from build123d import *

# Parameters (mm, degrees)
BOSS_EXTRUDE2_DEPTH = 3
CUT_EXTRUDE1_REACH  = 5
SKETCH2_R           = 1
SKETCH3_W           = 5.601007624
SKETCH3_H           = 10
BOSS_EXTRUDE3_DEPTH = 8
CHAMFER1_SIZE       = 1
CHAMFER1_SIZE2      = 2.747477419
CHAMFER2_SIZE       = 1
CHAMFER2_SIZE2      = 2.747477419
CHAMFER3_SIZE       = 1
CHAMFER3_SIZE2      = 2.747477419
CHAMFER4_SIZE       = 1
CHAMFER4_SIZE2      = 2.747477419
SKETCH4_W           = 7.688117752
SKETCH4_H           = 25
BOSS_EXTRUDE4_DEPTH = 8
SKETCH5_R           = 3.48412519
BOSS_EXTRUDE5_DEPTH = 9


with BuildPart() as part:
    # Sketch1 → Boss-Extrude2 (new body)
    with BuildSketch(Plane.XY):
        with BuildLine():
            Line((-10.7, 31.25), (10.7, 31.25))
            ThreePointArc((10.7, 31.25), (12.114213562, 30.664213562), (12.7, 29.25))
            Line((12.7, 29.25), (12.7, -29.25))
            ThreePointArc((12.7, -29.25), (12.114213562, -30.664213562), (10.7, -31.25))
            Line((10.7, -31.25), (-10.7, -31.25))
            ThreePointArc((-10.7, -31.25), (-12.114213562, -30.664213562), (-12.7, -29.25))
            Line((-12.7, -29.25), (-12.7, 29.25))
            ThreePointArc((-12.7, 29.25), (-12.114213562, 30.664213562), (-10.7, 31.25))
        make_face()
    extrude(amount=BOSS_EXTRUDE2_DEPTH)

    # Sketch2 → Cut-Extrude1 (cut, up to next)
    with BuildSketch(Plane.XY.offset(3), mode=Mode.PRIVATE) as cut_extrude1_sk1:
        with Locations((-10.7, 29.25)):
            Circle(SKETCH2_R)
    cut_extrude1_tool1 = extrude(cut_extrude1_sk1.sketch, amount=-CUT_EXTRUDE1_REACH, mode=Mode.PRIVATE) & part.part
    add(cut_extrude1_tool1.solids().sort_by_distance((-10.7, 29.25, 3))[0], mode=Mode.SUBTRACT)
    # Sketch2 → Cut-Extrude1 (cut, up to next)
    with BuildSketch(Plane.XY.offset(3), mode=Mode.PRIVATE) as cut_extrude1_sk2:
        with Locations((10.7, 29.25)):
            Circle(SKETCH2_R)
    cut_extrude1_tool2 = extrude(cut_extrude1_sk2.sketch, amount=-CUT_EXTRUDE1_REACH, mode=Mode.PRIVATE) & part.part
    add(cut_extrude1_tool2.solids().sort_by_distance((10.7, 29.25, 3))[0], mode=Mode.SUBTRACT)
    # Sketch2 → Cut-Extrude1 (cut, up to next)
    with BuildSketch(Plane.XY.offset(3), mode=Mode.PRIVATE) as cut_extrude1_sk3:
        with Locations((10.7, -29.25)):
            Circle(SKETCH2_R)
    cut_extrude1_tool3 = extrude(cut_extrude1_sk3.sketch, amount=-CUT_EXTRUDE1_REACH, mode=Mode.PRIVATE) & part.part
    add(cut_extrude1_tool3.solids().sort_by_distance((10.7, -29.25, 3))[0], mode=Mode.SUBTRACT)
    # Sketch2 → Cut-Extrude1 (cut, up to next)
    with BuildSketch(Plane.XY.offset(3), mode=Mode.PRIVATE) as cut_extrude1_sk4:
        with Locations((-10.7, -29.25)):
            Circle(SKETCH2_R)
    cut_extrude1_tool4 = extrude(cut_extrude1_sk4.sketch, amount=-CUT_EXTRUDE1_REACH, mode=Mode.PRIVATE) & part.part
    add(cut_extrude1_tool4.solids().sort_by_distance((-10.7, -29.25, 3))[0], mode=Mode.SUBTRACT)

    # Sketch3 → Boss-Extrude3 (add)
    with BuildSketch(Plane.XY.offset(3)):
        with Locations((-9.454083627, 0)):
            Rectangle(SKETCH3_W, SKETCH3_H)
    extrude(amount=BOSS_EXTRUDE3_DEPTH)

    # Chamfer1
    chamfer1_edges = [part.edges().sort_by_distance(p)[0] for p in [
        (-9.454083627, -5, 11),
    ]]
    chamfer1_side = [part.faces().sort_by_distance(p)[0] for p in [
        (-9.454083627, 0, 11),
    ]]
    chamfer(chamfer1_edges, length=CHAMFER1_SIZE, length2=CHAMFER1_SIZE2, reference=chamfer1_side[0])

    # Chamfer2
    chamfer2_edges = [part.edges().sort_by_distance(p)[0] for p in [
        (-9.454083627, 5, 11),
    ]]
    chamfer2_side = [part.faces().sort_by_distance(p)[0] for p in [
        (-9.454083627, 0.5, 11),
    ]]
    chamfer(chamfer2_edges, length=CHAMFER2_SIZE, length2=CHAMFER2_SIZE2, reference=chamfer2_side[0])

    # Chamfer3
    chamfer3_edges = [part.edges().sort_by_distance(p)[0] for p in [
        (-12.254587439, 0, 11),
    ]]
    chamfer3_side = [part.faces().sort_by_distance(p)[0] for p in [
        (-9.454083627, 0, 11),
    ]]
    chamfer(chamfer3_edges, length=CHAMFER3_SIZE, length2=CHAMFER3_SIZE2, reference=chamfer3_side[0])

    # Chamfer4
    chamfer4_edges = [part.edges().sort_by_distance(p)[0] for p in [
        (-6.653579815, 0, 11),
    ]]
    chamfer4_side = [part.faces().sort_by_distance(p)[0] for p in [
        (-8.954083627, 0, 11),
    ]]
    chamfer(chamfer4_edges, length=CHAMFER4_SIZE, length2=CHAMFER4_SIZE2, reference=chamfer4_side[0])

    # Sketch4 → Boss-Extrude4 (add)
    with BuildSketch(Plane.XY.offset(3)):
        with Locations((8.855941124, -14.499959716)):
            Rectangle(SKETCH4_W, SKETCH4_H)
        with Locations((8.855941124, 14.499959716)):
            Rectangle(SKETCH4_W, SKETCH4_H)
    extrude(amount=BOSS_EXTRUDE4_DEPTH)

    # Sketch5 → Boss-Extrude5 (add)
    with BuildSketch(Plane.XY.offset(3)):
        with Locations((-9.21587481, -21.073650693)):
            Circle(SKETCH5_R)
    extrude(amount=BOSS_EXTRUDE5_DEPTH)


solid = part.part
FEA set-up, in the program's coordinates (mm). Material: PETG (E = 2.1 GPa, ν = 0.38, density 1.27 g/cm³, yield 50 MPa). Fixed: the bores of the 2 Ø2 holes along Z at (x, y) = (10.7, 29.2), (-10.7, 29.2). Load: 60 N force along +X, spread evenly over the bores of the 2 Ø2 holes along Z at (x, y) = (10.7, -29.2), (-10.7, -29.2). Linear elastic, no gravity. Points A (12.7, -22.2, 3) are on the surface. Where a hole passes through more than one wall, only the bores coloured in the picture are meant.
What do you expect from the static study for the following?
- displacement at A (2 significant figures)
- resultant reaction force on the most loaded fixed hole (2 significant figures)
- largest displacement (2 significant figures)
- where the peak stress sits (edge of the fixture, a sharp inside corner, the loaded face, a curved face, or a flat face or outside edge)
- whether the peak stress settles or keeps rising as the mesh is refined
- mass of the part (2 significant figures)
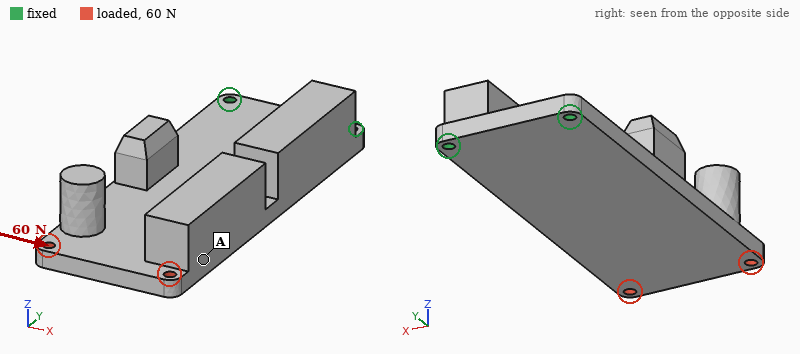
0.49 mm
170 N
0.66 mm
edge of the fixture
keeps rising
11 g
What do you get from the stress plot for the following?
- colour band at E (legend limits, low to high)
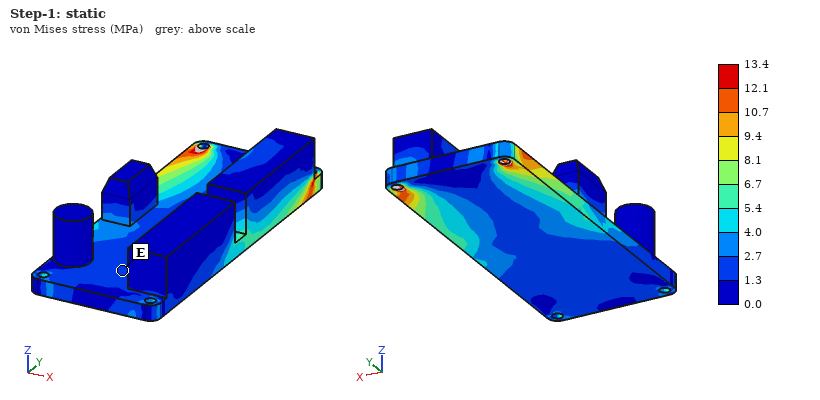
1.3 to 2.7 MPa
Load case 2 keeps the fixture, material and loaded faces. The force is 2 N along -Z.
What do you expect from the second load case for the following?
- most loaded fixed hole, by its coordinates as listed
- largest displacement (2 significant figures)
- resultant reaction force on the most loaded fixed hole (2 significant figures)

(-10.7, 29.2)
0.68 mm
1.5 N
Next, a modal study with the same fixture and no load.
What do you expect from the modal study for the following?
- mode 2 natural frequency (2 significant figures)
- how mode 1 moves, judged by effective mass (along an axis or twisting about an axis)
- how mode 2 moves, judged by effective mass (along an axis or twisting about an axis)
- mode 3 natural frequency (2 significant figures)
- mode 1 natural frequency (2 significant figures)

730 Hz
along Z
along X
990 Hz
160 Hz
